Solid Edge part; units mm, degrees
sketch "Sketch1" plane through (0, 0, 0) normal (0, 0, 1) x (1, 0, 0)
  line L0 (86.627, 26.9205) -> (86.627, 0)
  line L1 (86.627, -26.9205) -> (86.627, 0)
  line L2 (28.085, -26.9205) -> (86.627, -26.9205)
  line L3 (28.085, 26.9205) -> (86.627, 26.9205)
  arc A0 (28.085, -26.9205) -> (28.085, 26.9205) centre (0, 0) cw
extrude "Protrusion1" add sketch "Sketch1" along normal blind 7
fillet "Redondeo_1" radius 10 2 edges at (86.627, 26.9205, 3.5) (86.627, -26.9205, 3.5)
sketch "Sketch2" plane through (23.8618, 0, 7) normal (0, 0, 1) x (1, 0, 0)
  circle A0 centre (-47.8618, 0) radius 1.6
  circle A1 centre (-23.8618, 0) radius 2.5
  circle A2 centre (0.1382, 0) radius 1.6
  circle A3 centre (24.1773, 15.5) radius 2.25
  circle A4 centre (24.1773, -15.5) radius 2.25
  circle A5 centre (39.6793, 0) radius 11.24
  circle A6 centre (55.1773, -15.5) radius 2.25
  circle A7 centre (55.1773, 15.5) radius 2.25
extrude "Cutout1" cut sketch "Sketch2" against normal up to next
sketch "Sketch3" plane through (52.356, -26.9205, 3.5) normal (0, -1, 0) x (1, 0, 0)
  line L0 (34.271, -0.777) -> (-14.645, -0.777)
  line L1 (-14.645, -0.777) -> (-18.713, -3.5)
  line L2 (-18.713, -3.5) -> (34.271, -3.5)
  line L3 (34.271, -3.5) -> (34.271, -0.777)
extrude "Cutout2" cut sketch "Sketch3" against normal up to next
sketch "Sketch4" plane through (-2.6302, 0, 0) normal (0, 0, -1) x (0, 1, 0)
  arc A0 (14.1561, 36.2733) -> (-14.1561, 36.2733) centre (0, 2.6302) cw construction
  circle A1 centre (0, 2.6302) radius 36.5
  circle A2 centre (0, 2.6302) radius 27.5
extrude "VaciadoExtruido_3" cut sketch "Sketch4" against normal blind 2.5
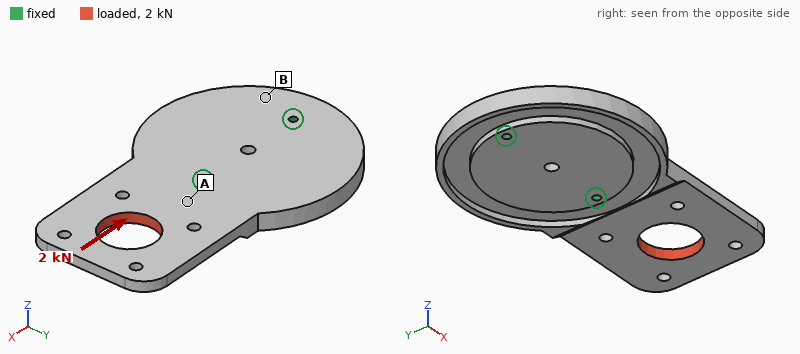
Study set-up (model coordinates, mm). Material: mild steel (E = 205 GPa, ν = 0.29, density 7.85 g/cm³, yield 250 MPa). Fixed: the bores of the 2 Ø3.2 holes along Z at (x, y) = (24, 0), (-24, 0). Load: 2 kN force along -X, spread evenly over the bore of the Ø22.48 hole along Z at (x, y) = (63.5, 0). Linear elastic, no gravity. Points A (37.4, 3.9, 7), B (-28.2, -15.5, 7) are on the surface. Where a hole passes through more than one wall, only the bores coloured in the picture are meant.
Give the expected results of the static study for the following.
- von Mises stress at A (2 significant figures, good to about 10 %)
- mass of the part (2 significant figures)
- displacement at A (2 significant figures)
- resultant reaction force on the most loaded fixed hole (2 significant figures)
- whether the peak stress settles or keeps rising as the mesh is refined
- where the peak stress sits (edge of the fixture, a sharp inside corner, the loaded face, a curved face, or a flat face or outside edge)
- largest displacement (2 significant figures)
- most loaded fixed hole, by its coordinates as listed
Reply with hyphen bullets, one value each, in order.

- 12 MPa
- 300 g
- 1.6 µm
- 1.4 kN
- keeps rising
- edge of the fixture
- 7.8 µm
- (24, 0)
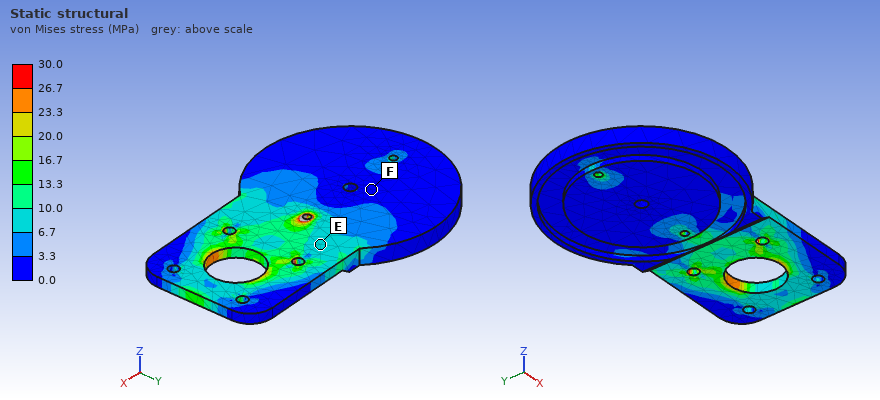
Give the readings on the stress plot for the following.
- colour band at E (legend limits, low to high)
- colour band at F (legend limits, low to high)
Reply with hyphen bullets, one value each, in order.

- 6.7 to 10.0 MPa
- 0.0 to 3.3 MPa
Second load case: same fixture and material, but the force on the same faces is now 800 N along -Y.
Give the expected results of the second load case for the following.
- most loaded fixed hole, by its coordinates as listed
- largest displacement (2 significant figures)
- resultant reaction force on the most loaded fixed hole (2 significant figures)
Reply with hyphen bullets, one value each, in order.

- (24, 0)
- 11 µm
- 1.4 kN
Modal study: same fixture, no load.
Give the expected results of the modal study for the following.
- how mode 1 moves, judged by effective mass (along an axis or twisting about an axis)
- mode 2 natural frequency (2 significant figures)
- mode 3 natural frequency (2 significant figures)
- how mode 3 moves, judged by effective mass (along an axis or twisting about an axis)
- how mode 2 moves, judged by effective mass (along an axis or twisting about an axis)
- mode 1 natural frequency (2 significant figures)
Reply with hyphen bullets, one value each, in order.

- along Z
- 2100 Hz
- 3300 Hz
- twisting about X
- twisting about X
- 1000 Hz
